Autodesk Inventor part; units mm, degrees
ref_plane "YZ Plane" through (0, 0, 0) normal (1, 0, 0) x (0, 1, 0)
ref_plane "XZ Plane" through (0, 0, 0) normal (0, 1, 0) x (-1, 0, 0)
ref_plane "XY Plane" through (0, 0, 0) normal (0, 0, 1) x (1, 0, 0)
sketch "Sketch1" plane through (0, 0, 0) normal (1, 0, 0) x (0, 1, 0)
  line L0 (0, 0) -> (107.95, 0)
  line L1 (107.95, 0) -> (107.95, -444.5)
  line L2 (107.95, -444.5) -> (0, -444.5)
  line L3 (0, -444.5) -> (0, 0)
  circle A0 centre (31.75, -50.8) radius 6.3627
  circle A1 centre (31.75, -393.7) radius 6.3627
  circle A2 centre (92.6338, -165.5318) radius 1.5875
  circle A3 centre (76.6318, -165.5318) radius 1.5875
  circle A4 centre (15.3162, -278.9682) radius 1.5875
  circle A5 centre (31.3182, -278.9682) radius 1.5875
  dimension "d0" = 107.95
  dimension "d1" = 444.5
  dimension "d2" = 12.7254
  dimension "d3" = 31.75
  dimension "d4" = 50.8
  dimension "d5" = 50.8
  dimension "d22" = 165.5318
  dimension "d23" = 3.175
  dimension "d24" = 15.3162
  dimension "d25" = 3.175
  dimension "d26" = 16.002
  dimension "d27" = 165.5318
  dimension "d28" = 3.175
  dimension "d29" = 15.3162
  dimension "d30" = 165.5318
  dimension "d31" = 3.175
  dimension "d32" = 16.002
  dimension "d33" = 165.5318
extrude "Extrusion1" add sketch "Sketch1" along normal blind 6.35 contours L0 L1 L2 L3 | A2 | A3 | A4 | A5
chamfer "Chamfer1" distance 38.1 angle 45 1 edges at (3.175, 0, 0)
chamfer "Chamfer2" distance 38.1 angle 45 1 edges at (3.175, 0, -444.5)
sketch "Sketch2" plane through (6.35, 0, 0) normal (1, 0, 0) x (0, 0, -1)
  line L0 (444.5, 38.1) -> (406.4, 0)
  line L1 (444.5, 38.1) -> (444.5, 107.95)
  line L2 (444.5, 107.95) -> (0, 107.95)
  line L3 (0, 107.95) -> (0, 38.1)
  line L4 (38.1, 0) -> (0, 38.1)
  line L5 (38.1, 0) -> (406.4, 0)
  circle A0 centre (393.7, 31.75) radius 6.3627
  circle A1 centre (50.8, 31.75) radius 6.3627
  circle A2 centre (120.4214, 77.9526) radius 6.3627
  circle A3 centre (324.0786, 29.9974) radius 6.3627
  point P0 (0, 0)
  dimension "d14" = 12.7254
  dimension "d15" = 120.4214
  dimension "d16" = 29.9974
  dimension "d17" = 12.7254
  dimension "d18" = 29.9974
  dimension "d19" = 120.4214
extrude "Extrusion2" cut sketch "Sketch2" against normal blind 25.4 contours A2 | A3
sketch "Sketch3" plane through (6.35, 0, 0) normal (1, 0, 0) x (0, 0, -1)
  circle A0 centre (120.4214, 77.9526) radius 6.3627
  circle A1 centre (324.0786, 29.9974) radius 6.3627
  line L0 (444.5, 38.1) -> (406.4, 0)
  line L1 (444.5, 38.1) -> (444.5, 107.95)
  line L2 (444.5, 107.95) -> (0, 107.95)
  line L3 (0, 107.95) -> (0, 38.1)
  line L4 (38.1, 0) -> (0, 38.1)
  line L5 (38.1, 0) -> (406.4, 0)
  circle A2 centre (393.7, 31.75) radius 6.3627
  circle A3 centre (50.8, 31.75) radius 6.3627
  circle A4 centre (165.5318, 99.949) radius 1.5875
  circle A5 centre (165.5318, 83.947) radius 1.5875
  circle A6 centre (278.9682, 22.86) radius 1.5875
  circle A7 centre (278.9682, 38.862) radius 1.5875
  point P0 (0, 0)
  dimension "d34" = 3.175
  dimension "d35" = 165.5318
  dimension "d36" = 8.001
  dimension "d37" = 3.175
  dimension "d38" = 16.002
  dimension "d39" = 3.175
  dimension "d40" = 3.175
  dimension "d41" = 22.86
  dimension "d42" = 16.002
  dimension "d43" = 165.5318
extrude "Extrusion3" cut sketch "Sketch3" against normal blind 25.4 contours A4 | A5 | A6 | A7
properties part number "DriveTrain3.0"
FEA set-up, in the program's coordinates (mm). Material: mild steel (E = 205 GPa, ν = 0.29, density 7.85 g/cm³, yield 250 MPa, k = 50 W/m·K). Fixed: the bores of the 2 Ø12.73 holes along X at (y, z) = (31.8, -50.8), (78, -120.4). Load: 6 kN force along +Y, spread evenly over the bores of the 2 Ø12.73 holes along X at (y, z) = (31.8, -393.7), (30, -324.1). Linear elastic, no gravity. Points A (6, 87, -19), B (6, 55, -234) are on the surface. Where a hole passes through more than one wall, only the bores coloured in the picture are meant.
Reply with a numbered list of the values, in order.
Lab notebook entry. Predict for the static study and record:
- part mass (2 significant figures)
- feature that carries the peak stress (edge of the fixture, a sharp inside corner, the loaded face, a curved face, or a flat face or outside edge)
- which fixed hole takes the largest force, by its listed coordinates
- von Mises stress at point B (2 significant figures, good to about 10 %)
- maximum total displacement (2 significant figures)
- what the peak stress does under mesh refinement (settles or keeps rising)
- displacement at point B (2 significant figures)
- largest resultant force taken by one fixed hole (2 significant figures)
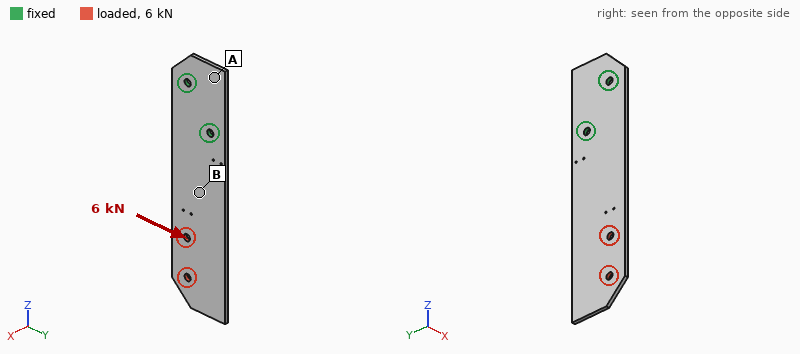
1. 2.3 kg
2. edge of the fixture
3. (78, -120.4)
4. 23 MPa
5. 0.49 mm
6. keeps rising
7. 0.13 mm
8. 21 kN
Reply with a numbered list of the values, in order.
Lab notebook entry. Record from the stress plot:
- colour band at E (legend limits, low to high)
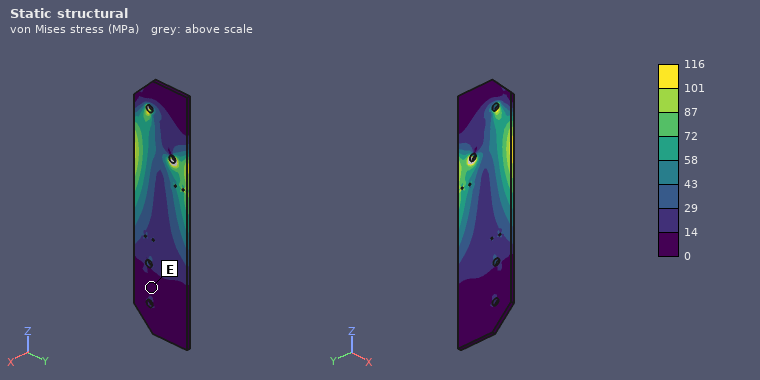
1. 0 to 14 MPa
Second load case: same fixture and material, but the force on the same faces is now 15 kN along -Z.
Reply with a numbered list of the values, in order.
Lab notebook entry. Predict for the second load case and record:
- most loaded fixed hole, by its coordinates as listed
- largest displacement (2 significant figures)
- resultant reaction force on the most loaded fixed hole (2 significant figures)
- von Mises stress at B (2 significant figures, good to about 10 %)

1. (31.8, -50.8)
2. 0.19 mm
3. 9.8 kN
4. 21 MPa
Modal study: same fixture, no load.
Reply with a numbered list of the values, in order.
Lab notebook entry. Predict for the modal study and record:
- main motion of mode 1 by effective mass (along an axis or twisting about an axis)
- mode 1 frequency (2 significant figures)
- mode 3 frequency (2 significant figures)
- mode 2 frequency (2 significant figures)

1. along X
2. 51 Hz
3. 340 Hz
4. 270 Hz
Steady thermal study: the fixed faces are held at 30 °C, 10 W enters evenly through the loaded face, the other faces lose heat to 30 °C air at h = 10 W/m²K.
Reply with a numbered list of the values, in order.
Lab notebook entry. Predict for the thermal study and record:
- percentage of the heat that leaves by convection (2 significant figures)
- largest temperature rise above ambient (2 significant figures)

1. 84 %
2. 25 K
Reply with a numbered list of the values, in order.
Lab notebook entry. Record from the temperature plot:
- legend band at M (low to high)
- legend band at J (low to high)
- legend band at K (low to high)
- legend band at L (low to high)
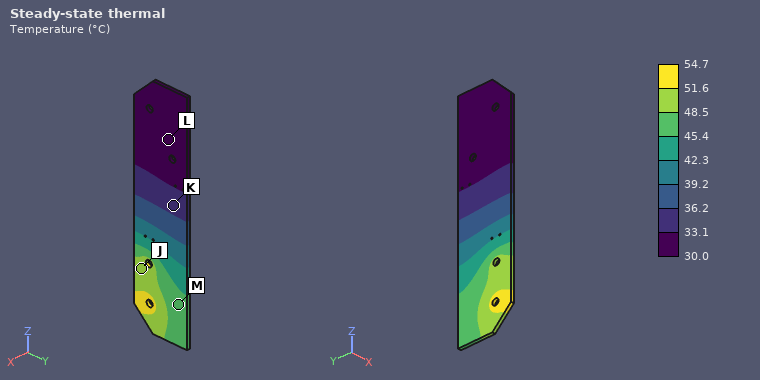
1. 45.4 to 48.5 °C
2. 48.5 to 51.6 °C
3. 33.1 to 36.2 °C
4. 30.0 to 33.1 °C
